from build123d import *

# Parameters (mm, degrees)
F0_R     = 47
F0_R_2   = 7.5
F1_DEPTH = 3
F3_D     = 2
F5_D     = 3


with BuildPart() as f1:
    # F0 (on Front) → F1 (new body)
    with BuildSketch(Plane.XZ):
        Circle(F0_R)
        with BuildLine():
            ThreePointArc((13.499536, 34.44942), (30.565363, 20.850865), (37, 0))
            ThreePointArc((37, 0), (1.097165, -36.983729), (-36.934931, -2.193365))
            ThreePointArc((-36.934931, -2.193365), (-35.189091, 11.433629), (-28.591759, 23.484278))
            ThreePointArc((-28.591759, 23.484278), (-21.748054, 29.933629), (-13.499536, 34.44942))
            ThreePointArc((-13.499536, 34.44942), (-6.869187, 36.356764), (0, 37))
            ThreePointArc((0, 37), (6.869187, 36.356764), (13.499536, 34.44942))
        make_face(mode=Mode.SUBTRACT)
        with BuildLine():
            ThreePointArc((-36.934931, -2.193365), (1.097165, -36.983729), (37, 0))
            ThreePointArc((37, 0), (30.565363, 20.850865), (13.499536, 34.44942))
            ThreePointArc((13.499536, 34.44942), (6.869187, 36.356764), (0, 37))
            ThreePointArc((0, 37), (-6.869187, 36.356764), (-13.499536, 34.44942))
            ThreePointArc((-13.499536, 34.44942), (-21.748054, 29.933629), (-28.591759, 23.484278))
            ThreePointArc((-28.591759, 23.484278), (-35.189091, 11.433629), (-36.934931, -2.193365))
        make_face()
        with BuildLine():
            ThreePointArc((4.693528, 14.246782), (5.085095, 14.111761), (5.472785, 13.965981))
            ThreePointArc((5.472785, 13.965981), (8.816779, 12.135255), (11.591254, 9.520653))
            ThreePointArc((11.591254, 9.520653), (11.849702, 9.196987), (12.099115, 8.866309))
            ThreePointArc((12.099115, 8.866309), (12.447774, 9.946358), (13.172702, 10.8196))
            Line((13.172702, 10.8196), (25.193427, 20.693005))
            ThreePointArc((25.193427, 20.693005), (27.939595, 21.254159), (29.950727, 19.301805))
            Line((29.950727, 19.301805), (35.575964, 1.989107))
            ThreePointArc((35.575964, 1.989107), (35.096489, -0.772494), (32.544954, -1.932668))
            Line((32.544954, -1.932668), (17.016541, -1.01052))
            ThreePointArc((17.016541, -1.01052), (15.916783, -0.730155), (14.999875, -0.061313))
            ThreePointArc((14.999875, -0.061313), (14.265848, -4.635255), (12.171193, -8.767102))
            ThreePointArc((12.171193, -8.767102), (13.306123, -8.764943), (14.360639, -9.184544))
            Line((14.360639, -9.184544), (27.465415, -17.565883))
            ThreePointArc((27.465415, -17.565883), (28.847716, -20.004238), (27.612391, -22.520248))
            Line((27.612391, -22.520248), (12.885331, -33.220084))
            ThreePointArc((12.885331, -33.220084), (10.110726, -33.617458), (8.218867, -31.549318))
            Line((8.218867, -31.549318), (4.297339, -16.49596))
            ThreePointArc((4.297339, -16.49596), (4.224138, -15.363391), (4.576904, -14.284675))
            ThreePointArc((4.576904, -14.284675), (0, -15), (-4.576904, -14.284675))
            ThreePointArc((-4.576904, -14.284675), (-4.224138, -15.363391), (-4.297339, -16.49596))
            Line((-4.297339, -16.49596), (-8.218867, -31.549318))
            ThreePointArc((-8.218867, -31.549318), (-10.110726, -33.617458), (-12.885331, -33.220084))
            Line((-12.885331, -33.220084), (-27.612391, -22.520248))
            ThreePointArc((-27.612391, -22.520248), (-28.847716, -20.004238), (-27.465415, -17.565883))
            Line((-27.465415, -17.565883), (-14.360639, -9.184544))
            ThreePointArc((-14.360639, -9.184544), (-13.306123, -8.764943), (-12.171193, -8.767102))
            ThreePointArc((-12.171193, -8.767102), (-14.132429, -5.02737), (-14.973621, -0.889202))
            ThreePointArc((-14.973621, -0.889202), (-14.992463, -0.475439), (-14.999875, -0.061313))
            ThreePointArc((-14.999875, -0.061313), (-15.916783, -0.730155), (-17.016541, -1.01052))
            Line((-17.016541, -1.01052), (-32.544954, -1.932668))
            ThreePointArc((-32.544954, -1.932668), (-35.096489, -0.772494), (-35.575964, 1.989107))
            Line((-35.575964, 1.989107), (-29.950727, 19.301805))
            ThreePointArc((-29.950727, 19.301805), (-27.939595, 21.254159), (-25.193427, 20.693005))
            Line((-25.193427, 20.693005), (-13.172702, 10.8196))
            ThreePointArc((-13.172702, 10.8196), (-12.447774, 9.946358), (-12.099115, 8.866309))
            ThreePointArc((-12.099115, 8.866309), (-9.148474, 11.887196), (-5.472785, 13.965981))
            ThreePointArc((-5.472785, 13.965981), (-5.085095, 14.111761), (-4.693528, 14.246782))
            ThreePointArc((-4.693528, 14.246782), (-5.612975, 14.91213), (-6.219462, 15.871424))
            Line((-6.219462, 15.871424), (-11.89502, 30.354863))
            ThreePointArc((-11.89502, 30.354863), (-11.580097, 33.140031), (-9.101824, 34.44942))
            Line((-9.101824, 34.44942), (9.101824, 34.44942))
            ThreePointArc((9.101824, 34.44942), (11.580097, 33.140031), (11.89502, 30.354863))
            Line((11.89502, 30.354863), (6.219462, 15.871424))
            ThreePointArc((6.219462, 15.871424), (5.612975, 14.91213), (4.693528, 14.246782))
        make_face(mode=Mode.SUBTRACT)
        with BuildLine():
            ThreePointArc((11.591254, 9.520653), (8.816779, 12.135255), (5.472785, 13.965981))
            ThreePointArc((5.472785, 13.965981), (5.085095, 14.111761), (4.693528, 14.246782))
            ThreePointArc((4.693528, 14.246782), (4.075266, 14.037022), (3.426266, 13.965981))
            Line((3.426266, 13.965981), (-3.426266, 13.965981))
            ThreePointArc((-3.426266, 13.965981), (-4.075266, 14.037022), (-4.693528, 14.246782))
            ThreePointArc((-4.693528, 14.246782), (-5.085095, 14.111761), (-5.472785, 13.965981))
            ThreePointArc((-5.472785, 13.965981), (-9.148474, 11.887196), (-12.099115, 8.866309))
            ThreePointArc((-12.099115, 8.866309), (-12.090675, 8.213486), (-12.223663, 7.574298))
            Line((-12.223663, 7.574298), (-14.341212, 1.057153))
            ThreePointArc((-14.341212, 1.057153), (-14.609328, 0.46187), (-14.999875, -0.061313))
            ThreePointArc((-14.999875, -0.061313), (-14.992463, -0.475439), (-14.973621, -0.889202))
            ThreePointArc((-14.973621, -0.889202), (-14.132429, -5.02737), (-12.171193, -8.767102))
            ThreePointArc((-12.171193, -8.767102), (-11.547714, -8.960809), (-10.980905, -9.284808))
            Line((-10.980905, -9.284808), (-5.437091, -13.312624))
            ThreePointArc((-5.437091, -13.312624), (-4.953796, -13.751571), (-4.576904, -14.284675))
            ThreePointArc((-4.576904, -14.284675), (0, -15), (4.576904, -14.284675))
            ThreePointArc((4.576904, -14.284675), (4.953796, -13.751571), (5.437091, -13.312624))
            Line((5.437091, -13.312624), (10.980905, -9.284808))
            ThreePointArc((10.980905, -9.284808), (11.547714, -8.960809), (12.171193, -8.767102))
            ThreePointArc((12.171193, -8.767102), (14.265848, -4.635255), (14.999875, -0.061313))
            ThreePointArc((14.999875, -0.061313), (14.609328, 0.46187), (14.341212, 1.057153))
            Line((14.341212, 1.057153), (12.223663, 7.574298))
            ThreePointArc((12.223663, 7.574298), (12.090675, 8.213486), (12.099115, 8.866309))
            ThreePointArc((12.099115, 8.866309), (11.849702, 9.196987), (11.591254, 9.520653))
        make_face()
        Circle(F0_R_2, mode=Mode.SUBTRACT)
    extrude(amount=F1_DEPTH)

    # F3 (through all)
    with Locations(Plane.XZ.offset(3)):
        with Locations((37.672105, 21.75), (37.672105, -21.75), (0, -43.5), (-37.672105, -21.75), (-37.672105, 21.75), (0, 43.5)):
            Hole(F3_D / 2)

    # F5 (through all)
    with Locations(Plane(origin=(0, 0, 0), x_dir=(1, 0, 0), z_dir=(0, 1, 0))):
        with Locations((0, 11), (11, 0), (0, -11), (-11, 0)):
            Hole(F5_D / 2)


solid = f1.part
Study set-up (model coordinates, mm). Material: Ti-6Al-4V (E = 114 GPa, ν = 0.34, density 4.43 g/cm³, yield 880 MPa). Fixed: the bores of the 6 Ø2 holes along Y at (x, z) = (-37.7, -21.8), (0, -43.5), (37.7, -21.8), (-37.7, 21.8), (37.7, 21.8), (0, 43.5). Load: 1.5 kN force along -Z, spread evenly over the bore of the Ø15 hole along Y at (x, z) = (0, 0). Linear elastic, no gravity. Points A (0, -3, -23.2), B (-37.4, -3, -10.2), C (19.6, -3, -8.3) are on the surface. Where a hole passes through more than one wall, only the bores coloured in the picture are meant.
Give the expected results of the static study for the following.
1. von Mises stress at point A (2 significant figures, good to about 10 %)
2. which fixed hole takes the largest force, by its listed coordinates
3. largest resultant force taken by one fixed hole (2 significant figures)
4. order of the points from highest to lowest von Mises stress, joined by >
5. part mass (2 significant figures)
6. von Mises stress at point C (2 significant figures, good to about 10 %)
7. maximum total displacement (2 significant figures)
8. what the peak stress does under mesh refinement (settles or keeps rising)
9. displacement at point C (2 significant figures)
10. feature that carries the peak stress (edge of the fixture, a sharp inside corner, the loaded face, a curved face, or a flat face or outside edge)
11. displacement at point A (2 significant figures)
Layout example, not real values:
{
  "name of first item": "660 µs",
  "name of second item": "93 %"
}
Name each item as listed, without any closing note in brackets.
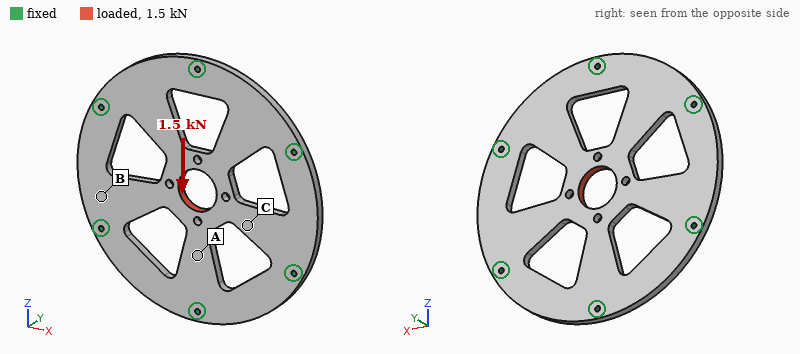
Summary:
{
  "von Mises stress at point A": "17 MPa",
  "which fixed hole takes the largest force, by its listed coordinates": "(0, -43.5)",
  "largest resultant force taken by one fixed hole": "520 N",
  "order of the points from highest to lowest von Mises stress, joined by >": "A > C > B",
  "part mass": "64 g",
  "von Mises stress at point C": "11 MPa",
  "maximum total displacement": "7.5 µm",
  "what the peak stress does under mesh refinement": "keeps rising",
  "displacement at point C": "3.1 µm",
  "feature that carries the peak stress": "edge of the fixture",
  "displacement at point A": "3.1 µm"
}
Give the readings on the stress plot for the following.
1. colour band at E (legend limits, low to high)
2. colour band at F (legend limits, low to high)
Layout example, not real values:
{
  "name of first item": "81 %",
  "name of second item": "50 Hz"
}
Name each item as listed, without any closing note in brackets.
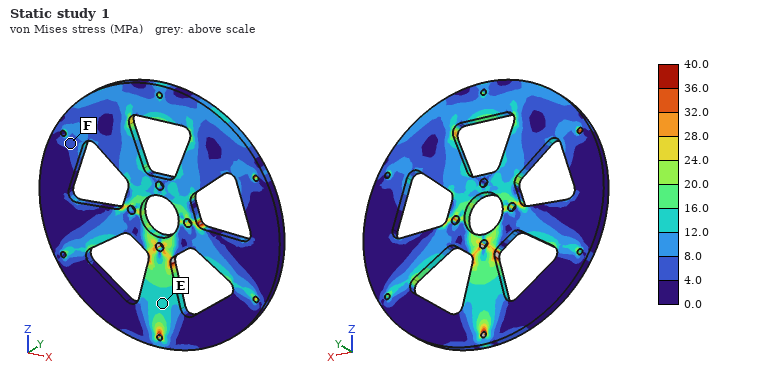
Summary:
{
  "colour band at E": "12.0 to 16.0 MPa",
  "colour band at F": "4.0 to 8.0 MPa"
}
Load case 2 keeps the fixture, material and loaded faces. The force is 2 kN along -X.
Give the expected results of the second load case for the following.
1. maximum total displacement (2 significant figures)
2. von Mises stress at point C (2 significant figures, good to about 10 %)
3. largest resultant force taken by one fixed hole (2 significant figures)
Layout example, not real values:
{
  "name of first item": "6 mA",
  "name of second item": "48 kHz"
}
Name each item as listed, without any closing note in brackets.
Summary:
{
  "maximum total displacement": "10 µm",
  "von Mises stress at point C": "22 MPa",
  "largest resultant force taken by one fixed hole": "500 N"
}
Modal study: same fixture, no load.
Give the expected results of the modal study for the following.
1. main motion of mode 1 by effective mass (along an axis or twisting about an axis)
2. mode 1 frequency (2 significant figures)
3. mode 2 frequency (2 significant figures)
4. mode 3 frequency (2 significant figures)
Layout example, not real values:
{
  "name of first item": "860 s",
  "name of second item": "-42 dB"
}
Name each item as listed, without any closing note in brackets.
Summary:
{
  "main motion of mode 1 by effective mass": "along Y",
  "mode 1 frequency": "2800 Hz",
  "mode 2 frequency": "5800 Hz",
  "mode 3 frequency": "5800 Hz"
}
